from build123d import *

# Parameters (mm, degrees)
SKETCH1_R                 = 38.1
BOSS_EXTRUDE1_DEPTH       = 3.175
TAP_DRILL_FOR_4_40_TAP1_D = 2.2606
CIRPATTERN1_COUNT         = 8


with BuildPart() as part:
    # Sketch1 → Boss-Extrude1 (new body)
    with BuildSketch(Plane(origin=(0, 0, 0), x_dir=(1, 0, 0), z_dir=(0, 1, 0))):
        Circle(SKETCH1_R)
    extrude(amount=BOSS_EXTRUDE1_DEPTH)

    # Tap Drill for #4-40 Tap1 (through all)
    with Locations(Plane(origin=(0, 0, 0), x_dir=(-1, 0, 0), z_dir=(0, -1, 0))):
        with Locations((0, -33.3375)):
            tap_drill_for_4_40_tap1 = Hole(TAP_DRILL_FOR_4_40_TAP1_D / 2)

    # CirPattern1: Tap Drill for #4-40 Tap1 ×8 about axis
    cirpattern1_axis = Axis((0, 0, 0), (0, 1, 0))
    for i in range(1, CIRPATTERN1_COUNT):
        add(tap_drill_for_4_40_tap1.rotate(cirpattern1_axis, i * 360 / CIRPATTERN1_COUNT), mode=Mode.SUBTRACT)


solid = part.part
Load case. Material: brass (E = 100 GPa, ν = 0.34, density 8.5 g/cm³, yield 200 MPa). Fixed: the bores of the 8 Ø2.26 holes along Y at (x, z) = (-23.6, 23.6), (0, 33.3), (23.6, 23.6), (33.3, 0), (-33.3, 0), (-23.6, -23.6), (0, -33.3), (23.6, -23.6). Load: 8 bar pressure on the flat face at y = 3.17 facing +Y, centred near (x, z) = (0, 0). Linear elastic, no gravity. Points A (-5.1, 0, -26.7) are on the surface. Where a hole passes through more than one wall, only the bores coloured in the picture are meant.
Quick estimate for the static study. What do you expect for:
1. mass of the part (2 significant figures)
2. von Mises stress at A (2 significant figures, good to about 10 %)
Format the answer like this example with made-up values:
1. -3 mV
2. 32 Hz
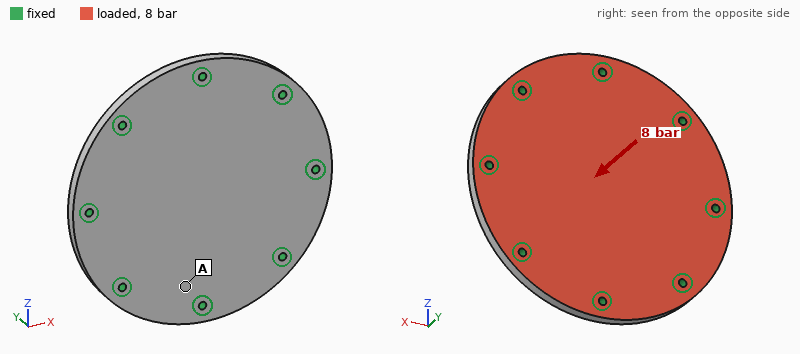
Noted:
1. 120 g
2. 29 MPa
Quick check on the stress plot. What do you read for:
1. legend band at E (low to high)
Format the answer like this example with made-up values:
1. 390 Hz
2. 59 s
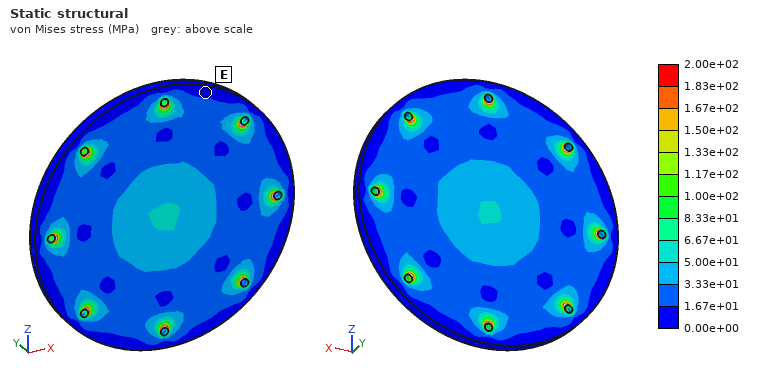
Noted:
1. 0.00e+00 to 1.67e+01 MPa
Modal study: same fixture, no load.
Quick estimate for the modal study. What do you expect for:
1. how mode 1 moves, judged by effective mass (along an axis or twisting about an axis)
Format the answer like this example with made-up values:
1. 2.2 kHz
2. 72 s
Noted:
1. along Y
